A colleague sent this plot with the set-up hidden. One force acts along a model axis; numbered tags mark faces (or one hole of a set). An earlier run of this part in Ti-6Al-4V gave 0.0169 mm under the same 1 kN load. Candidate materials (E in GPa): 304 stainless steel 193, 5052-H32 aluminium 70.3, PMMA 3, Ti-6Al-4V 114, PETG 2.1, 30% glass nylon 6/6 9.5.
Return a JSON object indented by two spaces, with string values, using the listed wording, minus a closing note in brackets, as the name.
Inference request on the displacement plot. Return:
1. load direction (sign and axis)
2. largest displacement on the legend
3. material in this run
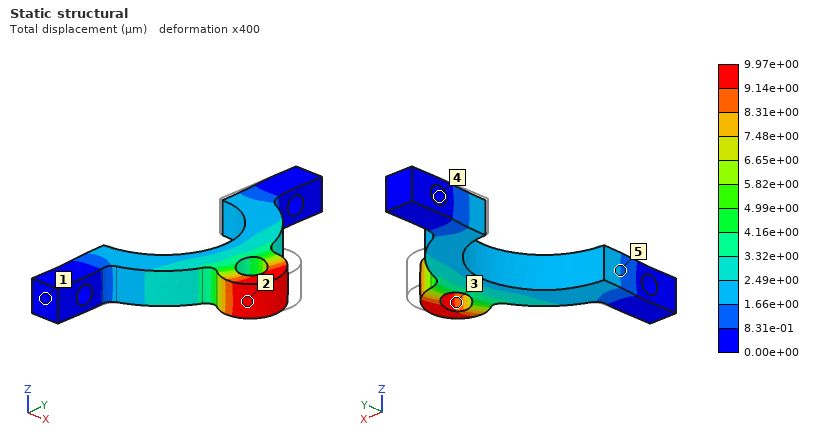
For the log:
{
  "load direction": "-Y",
  "largest displacement on the legend": "9.97e+00 µm",
  "material in this run": "304 stainless steel"
}
